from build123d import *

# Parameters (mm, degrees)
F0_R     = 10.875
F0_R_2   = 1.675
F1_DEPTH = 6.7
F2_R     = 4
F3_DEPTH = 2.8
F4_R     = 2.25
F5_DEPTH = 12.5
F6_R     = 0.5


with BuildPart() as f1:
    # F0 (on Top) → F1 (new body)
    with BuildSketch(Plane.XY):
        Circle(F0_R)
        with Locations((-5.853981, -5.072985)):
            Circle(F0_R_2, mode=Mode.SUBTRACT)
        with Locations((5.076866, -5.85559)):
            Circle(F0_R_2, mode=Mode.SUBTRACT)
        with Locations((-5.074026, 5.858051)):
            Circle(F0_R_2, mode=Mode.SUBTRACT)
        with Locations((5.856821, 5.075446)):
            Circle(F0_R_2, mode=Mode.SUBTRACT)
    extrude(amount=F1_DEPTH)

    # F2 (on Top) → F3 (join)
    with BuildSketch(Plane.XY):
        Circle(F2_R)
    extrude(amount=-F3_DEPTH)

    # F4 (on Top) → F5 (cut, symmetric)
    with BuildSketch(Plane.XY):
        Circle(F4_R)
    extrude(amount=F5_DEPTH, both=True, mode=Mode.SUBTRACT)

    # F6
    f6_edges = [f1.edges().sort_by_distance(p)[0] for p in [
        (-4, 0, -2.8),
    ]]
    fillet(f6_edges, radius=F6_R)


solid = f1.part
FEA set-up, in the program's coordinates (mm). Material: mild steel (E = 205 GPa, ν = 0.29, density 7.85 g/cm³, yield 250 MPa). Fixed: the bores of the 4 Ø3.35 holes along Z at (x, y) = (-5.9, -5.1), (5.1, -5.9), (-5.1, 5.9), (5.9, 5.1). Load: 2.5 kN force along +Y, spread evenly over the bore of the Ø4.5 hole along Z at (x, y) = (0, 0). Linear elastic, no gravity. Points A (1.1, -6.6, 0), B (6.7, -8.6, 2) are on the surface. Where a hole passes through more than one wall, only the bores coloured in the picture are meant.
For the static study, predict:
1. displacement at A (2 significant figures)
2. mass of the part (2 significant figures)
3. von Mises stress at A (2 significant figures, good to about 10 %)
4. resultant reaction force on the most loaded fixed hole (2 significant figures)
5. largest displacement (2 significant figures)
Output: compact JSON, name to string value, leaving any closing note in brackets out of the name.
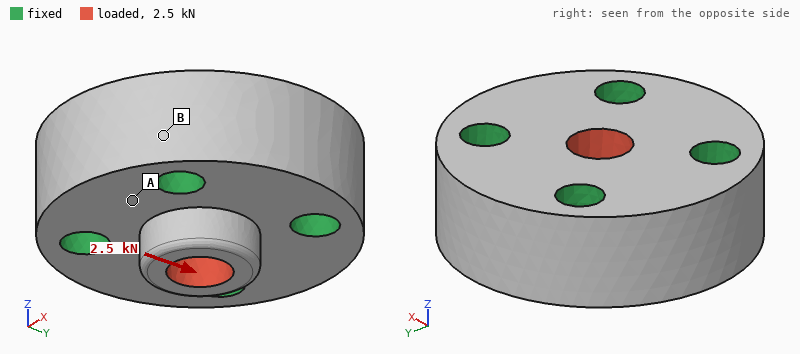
{"displacement at A": "0.32 µm", "mass of the part": "18 g", "von Mises stress at A": "11 MPa", "resultant reaction force on the most loaded fixed hole": "710 N", "largest displacement": "2.0 µm"}
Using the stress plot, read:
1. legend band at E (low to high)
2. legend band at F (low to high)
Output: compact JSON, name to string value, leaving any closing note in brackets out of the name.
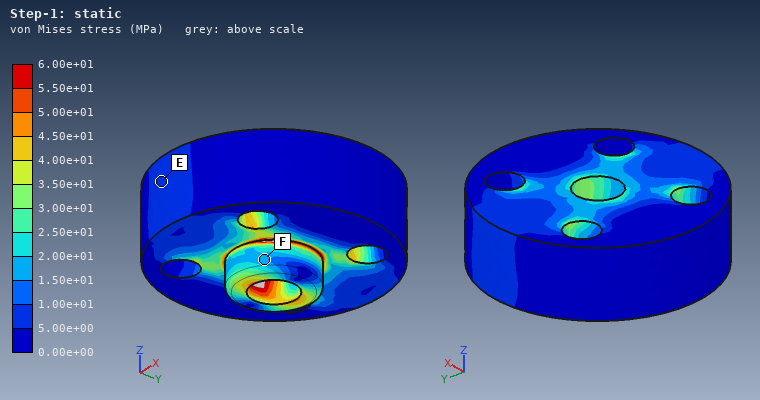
{"legend band at E": "5.00e+00 to 1.00e+01 MPa", "legend band at F": "1.50e+01 to 2.00e+01 MPa"}
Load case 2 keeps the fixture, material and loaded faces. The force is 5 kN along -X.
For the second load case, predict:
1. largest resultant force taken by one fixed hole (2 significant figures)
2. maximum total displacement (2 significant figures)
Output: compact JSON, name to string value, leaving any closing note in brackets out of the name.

{"largest resultant force taken by one fixed hole": "1.4 kN", "maximum total displacement": "4.0 µm"}
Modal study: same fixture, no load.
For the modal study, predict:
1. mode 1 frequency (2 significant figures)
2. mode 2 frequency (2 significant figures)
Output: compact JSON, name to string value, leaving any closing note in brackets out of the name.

{"mode 1 frequency": "120 kHz", "mode 2 frequency": "120 kHz"}
